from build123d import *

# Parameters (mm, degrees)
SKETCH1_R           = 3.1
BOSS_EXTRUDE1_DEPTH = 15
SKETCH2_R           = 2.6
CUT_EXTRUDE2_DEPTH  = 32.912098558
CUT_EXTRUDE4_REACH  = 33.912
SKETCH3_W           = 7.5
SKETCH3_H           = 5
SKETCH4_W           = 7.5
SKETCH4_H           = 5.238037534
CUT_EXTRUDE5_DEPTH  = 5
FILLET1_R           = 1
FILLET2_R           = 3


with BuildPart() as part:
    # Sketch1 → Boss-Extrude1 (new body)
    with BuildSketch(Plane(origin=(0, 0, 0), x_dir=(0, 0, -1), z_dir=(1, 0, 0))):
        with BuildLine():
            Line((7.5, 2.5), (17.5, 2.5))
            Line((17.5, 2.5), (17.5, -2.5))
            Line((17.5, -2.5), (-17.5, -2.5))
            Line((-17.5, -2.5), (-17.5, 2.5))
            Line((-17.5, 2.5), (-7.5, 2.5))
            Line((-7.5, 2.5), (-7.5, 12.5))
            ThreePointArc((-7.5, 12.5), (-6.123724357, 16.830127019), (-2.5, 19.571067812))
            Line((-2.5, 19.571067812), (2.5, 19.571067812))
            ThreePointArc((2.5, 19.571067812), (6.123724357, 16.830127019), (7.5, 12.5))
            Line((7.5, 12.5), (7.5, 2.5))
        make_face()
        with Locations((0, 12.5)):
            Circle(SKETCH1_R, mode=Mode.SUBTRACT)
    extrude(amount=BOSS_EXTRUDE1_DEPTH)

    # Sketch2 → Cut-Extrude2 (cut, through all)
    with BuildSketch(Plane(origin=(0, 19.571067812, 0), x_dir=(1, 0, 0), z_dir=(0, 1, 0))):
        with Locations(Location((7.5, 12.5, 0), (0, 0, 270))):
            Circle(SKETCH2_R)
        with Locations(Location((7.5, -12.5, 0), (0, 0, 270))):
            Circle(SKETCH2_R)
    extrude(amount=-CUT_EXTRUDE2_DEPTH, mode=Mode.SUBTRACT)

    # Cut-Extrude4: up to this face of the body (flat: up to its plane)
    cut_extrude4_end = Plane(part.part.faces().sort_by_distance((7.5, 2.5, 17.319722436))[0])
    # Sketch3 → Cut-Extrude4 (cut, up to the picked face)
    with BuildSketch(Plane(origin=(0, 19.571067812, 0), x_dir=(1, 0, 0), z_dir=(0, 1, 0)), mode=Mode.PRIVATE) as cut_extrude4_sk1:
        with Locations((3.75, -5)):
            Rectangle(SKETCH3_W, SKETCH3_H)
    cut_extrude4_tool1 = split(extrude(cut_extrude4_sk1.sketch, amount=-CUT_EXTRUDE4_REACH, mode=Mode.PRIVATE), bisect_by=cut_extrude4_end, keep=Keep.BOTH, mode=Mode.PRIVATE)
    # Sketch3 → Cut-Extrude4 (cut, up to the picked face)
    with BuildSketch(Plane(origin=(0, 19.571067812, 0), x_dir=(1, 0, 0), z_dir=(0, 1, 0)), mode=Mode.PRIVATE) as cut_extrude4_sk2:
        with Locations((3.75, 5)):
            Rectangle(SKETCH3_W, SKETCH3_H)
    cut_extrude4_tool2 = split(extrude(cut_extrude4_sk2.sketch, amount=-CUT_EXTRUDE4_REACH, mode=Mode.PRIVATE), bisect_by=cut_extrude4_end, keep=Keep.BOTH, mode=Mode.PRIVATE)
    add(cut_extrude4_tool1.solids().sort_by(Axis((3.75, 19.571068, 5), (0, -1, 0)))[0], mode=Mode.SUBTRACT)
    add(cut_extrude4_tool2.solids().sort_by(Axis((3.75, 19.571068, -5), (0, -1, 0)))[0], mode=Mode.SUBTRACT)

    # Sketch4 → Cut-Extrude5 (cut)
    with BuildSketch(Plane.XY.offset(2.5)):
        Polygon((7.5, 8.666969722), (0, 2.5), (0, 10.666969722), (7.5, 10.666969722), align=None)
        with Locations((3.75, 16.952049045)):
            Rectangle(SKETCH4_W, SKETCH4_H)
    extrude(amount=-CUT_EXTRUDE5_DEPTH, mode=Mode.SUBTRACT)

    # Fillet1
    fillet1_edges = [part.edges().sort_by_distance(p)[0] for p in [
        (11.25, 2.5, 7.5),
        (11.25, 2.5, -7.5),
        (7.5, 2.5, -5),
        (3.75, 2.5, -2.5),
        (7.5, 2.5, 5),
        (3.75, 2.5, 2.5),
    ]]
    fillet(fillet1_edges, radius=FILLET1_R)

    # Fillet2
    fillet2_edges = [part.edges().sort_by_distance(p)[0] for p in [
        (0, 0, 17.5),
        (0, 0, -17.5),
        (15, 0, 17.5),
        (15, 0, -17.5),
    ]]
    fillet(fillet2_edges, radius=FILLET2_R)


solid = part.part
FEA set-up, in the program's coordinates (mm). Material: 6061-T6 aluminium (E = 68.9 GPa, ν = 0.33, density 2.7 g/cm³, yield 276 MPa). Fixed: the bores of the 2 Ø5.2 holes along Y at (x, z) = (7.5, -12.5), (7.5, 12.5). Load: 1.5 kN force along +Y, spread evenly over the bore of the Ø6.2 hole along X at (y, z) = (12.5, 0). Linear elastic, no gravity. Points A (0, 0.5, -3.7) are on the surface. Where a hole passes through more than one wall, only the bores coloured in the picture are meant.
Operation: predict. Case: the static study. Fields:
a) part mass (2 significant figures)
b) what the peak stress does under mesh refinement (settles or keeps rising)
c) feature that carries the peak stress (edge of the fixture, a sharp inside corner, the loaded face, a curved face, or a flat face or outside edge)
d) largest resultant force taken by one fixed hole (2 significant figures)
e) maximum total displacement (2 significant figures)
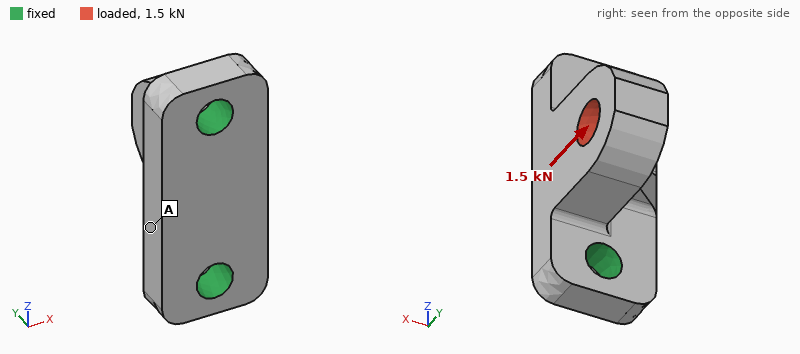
11 g
keeps rising
edge of the fixture
790 N
24 µm
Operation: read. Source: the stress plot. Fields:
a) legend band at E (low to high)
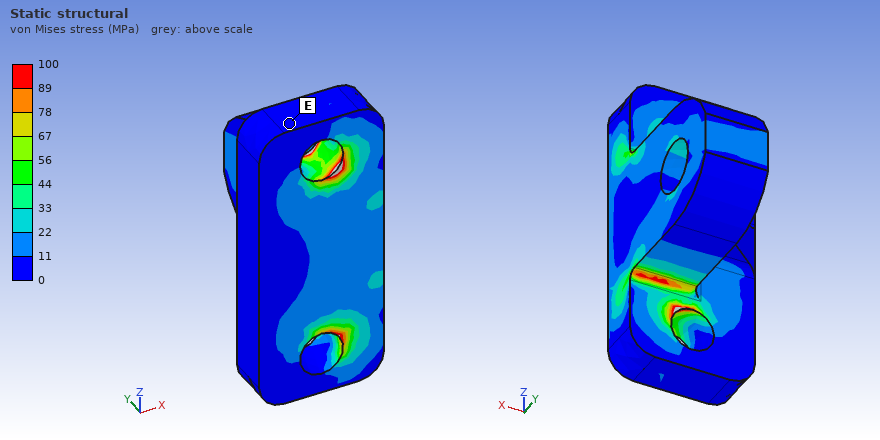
0 to 11 MPa
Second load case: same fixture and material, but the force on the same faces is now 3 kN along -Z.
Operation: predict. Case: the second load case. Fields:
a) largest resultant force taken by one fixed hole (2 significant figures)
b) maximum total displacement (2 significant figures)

2.5 kN
65 µm
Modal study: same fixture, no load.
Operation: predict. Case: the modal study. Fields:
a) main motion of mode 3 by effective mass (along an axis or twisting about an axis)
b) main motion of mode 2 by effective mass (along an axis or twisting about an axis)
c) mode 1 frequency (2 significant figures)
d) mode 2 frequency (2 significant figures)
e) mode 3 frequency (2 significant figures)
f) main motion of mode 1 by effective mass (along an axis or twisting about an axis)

along Y
along Z
12 kHz
22 kHz
30 kHz
along X
